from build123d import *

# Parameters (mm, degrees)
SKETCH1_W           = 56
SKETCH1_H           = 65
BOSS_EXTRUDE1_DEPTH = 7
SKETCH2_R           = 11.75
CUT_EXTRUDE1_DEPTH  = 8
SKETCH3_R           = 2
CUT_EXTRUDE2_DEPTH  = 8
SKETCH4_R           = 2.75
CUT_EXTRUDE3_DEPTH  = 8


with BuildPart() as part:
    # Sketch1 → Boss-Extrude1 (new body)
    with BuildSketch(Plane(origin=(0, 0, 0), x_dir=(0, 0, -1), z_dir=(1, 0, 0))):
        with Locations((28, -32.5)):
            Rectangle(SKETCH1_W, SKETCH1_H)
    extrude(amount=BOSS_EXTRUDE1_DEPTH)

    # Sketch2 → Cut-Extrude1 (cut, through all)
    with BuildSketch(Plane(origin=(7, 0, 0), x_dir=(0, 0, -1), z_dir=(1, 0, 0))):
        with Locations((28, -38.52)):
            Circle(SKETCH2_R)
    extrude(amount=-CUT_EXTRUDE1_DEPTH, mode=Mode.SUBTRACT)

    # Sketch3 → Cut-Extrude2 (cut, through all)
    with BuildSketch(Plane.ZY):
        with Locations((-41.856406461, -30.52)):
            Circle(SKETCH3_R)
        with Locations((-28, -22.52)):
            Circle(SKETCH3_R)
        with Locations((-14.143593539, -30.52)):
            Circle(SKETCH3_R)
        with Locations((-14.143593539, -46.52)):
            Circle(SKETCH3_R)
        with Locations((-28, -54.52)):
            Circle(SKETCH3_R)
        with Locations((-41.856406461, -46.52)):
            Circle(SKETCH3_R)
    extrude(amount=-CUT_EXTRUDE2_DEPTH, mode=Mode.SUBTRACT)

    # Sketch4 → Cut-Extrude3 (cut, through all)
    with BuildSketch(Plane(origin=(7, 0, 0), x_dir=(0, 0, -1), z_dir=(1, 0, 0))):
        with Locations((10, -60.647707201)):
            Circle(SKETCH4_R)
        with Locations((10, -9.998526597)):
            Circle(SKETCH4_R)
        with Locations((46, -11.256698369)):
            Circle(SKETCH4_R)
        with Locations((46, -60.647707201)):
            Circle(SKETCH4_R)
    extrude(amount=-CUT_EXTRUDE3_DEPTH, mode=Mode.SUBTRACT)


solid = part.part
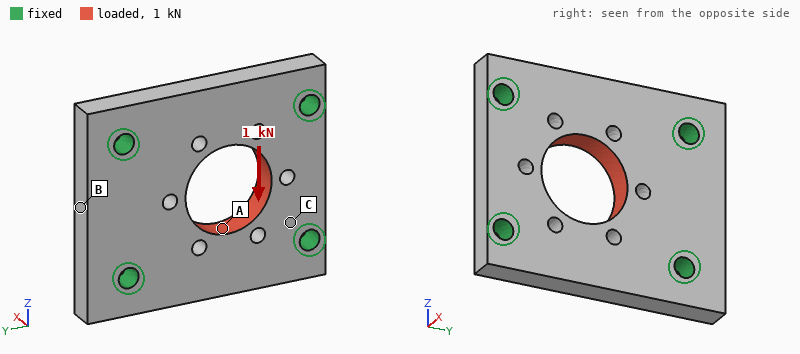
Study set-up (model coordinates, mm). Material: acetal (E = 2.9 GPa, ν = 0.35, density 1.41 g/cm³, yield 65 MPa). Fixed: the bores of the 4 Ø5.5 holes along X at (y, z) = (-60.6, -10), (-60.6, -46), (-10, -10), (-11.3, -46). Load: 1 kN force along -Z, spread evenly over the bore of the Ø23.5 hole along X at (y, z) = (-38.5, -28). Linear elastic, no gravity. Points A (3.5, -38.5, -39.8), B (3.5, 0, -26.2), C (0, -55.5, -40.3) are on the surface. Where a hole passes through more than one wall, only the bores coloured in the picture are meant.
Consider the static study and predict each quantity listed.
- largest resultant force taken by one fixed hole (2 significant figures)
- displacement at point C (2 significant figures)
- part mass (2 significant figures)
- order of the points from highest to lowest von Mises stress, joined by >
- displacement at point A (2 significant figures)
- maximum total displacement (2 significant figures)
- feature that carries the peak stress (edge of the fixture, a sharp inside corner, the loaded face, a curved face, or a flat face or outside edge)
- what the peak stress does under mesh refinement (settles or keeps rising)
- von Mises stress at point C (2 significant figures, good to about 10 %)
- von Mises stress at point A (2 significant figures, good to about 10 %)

280 N
9.9 µm
30 g
C > A > B
39 µm
41 µm
edge of the fixture
keeps rising
3.0 MPa
1.8 MPa
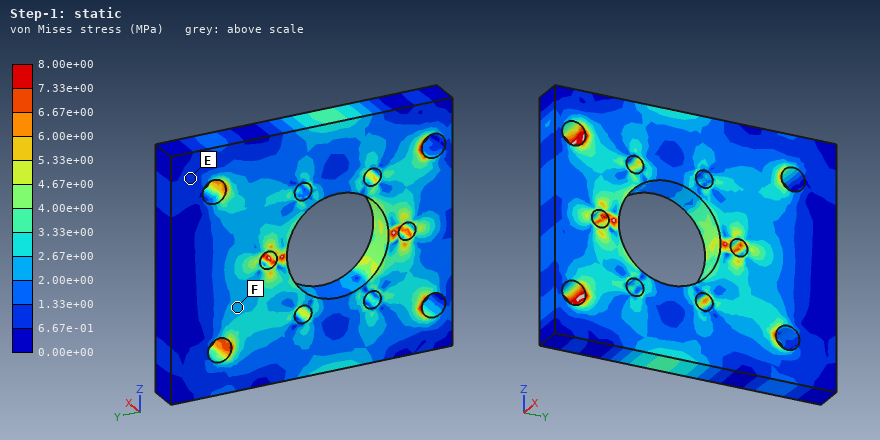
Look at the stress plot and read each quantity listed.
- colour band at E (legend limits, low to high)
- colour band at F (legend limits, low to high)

6.67e-01 to 1.33e+00 MPa
2.00e+00 to 2.67e+00 MPa
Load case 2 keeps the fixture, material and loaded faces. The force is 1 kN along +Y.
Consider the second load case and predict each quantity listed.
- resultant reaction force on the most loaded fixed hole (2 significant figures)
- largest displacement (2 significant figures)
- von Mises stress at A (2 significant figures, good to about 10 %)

280 N
30 µm
3.4 MPa
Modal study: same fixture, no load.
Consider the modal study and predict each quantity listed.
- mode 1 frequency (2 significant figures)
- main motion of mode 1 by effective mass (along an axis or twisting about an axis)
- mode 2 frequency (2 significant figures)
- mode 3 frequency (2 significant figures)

3700 Hz
along X
4100 Hz
5300 Hz
